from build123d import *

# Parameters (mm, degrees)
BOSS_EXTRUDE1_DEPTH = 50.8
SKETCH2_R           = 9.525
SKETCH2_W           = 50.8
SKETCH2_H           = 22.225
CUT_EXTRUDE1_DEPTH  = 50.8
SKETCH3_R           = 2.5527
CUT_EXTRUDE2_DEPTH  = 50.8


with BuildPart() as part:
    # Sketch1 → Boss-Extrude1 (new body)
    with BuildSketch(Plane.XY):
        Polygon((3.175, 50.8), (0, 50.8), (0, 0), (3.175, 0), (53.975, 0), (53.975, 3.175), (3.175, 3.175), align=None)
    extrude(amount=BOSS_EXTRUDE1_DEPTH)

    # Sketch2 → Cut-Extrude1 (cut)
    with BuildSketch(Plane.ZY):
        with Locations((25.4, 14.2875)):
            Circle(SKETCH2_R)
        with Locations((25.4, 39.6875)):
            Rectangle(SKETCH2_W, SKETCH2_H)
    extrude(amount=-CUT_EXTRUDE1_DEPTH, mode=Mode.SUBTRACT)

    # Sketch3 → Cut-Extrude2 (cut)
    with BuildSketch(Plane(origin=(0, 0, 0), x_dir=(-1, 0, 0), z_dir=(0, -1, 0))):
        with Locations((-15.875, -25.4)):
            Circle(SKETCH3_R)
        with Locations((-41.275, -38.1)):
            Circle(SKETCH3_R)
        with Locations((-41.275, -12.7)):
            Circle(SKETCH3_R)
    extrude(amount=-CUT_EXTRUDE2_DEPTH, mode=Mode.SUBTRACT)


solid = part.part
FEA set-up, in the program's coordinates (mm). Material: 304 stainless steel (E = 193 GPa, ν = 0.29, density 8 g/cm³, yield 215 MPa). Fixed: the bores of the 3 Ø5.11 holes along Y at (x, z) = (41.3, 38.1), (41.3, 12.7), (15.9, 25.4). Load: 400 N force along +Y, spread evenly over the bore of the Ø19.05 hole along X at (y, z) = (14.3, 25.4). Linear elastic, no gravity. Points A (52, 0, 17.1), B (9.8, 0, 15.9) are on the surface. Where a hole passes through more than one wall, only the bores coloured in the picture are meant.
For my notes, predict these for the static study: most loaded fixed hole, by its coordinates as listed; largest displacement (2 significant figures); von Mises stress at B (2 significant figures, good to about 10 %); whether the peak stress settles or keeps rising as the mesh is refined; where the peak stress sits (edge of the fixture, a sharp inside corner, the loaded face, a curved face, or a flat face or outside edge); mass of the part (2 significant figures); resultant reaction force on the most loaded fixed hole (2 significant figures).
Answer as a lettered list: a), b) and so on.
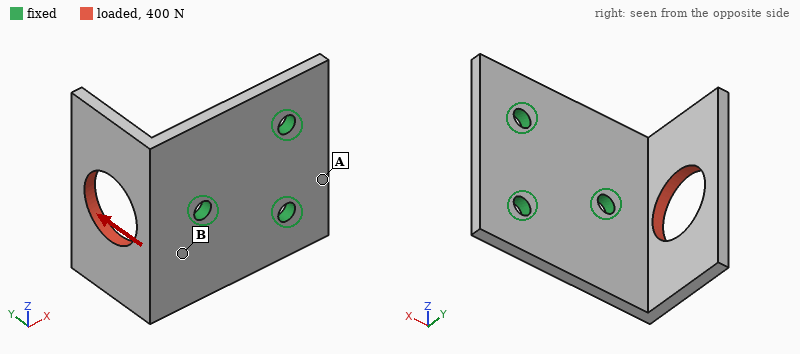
a) (15.9, 25.4)
b) 54 µm
c) 37 MPa
d) keeps rising
e) edge of the fixture
f) 94 g
g) 480 N
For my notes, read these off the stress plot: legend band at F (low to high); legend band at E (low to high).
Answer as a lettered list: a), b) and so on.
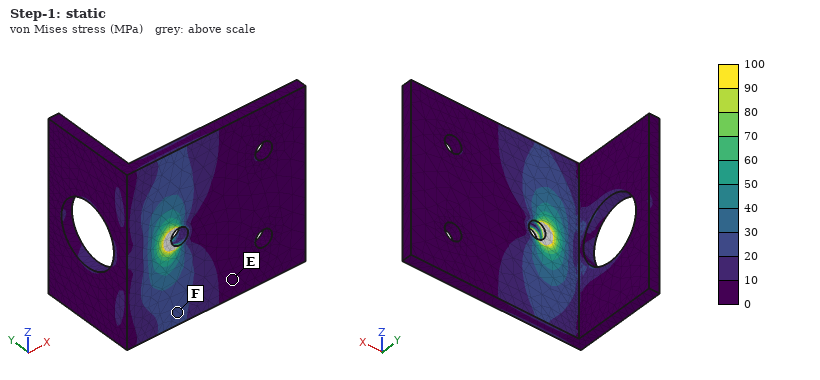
a) 20 to 30 MPa
b) 0 to 10 MPa
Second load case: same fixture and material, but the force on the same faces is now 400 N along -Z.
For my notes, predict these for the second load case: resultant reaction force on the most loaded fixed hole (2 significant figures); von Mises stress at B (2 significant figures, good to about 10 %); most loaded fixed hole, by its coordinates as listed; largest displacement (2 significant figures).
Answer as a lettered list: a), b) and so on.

a) 460 N
b) 20 MPa
c) (15.9, 25.4)
d) 68 µm
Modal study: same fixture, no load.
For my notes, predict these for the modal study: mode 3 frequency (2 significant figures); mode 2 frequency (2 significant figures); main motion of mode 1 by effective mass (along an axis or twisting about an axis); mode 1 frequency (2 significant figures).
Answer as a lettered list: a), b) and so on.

a) 4000 Hz
b) 2000 Hz
c) along X
d) 1900 Hz
